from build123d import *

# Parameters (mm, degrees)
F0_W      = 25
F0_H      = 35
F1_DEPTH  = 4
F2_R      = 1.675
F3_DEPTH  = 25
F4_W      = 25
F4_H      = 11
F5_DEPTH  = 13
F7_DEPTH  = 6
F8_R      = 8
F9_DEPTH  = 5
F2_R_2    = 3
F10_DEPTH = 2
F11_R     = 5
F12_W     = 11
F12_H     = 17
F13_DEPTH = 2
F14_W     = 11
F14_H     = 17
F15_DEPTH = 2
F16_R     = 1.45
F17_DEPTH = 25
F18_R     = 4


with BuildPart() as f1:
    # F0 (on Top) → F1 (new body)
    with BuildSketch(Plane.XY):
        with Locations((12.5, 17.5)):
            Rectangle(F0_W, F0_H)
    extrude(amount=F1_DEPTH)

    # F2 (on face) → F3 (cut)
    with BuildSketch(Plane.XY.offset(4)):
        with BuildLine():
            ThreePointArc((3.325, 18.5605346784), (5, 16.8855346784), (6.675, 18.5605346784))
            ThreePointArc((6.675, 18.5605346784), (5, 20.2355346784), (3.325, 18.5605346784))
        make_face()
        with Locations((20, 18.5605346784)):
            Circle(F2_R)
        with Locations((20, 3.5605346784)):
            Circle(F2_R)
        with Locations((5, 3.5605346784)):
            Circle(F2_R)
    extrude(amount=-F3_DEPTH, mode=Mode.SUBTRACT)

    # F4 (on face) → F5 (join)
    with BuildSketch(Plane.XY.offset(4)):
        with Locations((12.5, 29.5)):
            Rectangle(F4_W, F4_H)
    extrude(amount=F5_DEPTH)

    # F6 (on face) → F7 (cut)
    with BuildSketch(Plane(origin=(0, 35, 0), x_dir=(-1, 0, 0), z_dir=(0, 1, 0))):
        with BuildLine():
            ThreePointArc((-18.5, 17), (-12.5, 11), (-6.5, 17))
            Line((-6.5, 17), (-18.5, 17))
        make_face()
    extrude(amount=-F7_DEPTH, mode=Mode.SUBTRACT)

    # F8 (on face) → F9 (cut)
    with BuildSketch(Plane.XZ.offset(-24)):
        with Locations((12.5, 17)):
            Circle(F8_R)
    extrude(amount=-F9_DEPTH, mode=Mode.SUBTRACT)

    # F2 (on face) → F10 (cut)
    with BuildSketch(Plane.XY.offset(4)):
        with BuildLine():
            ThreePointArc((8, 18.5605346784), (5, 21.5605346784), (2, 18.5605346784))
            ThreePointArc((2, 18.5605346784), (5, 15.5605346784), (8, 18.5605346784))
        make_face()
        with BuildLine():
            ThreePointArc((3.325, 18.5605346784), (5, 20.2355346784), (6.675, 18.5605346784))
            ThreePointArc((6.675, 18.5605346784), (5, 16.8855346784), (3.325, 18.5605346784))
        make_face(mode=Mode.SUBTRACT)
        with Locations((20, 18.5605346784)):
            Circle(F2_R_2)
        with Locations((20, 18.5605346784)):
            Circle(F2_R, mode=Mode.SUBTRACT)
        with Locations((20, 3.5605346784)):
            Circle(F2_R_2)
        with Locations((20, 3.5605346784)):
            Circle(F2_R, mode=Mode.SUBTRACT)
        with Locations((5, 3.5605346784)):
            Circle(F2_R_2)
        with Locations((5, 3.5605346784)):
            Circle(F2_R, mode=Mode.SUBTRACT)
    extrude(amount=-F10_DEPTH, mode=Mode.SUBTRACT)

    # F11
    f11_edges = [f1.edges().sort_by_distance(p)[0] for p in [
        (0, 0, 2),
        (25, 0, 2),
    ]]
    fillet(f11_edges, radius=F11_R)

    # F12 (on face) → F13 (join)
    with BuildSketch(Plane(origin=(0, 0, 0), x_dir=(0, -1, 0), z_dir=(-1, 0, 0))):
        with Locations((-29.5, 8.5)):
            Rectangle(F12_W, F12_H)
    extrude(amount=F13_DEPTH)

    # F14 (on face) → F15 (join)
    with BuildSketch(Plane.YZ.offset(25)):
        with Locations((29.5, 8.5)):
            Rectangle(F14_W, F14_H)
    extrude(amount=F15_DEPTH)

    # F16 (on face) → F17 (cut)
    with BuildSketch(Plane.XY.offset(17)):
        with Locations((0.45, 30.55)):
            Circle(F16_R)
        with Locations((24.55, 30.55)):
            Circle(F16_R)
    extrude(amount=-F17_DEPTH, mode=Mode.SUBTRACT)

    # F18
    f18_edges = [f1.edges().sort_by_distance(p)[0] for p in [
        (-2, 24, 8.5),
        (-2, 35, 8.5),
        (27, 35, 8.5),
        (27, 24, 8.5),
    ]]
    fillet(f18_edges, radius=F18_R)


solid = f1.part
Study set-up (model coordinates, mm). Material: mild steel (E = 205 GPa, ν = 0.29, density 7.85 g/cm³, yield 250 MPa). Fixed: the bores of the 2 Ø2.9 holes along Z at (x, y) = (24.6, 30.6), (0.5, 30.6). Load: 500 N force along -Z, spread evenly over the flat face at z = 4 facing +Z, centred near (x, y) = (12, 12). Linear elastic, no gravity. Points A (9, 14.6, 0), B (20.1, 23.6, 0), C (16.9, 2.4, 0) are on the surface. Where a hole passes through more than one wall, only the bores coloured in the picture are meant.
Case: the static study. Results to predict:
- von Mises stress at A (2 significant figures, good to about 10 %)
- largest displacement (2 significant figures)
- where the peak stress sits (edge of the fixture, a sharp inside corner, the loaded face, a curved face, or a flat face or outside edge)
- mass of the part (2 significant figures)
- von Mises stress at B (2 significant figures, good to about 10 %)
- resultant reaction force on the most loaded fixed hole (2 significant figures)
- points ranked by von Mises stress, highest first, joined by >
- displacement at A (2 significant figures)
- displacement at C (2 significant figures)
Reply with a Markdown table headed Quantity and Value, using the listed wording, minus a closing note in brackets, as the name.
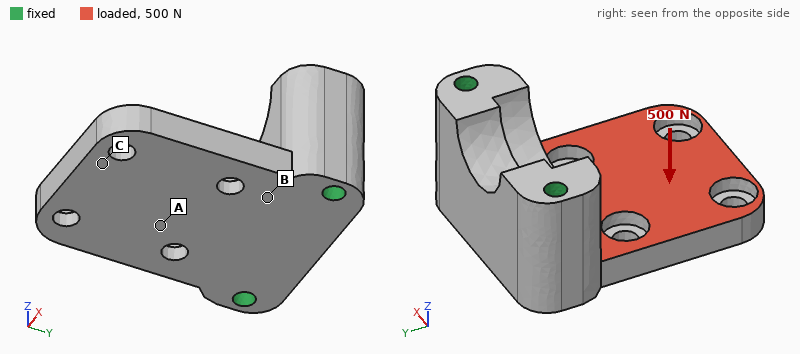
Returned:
| Quantity | Value |
|---|---|
| von Mises stress at A | 32 MPa |
| largest displacement | 53 µm |
| where the peak stress sits | the loaded face |
| mass of the part | 49 g |
| von Mises stress at B | 61 MPa |
| resultant reaction force on the most loaded fixed hole | 250 N |
| points ranked by von Mises stress, highest first, joined by > | B > A > C |
| displacement at A | 17 µm |
| displacement at C | 47 µm |
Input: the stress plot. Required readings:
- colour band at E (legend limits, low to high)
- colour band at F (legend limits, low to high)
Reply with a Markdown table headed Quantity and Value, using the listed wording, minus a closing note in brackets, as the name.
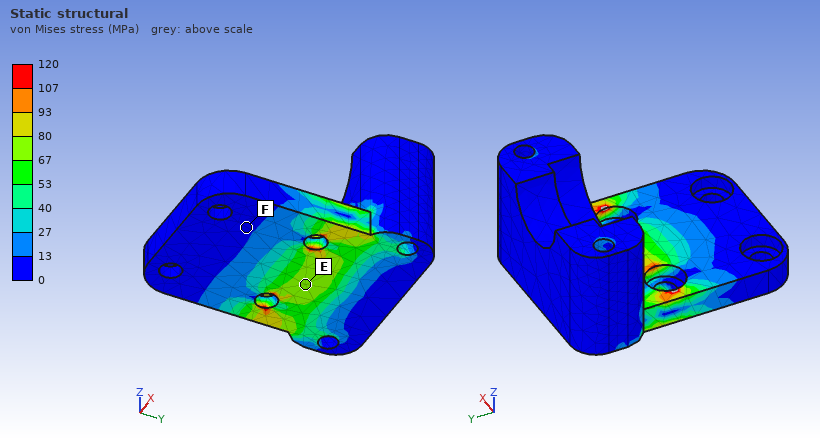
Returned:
| Quantity | Value |
|---|---|
| colour band at E | 67 to 80 MPa |
| colour band at F | 0 to 13 MPa |
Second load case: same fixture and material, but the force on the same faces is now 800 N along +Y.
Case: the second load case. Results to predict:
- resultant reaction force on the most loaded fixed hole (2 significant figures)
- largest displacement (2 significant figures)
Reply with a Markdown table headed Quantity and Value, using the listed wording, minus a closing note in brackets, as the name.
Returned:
| Quantity | Value |
|---|---|
| resultant reaction force on the most loaded fixed hole | 410 N |
| largest displacement | 17 µm |
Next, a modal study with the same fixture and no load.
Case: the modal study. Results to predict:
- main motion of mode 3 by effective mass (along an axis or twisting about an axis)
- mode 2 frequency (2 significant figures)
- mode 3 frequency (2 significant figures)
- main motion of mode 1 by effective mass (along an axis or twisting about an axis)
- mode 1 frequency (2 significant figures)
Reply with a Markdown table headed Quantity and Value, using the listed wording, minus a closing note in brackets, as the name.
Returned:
| Quantity | Value |
|---|---|
| main motion of mode 3 by effective mass | along X |
| mode 2 frequency | 12 kHz |
| mode 3 frequency | 18 kHz |
| main motion of mode 1 by effective mass | along Z |
| mode 1 frequency | 4800 Hz |
